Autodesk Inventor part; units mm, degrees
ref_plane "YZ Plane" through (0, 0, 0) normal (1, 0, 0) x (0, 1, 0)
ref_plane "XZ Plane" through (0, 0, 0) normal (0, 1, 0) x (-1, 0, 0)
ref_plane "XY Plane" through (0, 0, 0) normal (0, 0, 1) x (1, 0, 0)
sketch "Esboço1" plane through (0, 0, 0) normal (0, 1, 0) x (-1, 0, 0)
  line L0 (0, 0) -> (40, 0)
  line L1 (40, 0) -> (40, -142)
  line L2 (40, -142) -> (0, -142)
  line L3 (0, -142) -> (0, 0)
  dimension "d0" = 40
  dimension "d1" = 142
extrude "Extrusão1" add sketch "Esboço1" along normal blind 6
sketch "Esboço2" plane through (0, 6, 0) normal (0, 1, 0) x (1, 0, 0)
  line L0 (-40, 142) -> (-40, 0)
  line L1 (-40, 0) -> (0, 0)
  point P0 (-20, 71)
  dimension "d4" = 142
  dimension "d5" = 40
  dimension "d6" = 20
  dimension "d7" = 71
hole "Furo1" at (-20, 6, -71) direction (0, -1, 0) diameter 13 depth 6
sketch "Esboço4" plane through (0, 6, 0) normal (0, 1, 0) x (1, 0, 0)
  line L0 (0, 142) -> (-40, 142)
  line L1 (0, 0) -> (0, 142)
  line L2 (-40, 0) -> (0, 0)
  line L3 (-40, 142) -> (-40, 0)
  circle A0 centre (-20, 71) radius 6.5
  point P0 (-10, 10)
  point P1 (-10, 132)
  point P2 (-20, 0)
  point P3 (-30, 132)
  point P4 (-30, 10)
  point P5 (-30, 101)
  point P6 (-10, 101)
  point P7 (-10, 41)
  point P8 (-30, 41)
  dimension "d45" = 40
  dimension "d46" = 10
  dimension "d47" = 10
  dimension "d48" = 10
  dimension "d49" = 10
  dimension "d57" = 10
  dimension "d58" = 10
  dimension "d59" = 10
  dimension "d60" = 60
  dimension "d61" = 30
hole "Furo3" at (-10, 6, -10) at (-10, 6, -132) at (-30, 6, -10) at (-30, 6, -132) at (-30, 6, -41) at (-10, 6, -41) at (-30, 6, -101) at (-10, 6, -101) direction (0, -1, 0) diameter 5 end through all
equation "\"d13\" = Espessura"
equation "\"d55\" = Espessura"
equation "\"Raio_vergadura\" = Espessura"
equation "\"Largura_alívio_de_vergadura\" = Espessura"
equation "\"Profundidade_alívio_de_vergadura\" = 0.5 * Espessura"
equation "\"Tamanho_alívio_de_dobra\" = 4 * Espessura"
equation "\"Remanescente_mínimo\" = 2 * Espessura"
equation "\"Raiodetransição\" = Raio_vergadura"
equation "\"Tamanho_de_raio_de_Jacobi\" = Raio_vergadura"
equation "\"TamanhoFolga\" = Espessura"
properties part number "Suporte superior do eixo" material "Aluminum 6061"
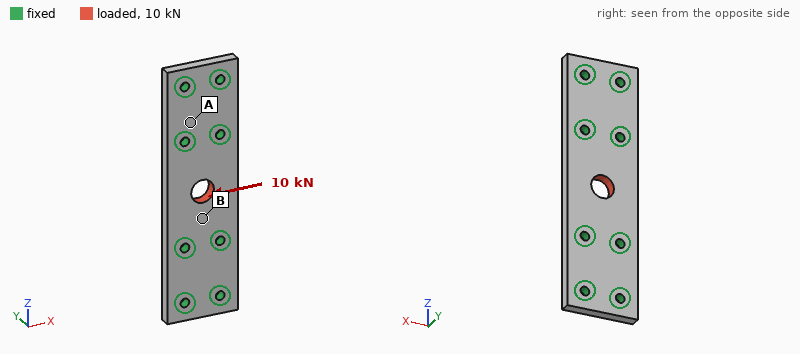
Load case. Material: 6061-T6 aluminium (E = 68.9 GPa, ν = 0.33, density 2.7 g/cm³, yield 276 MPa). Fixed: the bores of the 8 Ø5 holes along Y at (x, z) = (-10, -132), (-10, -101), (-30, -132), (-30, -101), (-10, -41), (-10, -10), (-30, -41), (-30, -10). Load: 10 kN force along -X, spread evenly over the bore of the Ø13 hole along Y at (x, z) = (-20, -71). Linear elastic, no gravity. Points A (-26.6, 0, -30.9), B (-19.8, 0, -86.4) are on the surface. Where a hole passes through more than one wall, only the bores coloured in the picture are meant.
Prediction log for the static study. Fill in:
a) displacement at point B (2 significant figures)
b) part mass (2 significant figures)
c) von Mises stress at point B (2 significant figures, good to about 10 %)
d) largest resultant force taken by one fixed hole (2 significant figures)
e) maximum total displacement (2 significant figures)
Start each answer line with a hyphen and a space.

- 17 µm
- 87 g
- 54 MPa
- 3.3 kN
- 33 µm
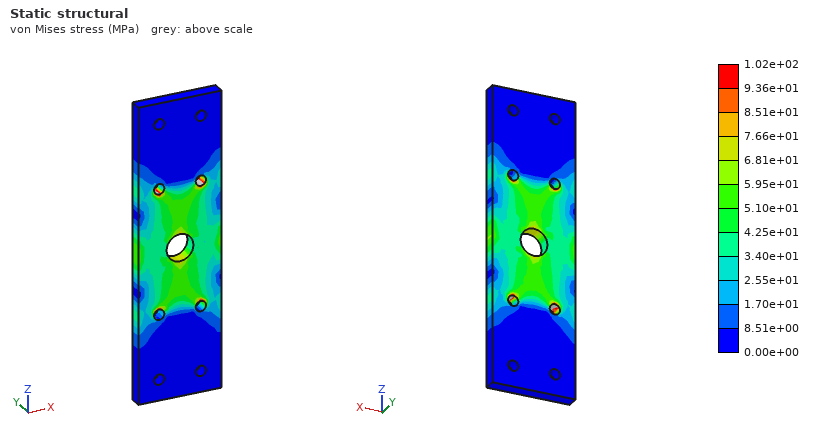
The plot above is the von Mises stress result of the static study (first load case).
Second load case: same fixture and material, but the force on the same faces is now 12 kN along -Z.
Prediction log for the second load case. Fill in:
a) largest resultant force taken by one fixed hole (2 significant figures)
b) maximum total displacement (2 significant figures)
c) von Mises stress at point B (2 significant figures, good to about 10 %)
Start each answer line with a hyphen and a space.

- 2.8 kN
- 15 µm
- 41 MPa
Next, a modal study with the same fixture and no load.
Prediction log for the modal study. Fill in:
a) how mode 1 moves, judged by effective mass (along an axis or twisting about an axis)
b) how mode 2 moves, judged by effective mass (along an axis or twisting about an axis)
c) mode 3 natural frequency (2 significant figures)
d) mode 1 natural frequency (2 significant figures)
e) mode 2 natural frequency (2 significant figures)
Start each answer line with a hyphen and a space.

- along Y
- twisting about Z
- 21 kHz
- 8500 Hz
- 11 kHz
